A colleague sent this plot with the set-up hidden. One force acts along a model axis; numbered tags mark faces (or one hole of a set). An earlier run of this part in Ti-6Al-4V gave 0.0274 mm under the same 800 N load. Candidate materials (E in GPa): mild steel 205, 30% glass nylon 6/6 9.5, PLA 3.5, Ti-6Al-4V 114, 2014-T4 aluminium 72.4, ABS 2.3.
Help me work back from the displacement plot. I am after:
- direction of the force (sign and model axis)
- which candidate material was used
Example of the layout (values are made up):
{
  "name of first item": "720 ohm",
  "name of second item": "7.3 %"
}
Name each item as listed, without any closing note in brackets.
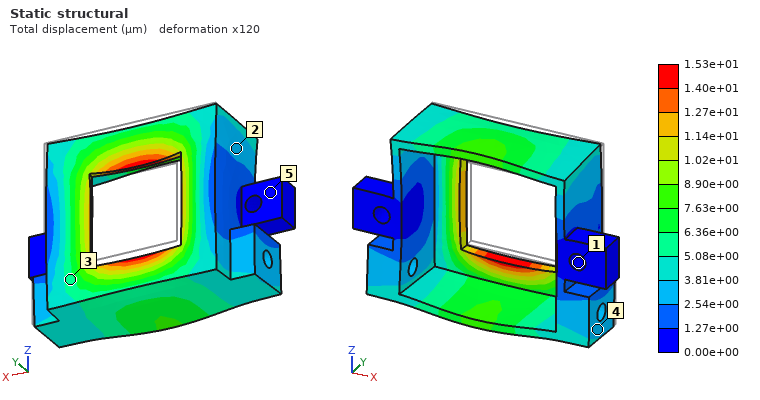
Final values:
{
  "direction of the force": "-Y",
  "which candidate material was used": "mild steel"
}
